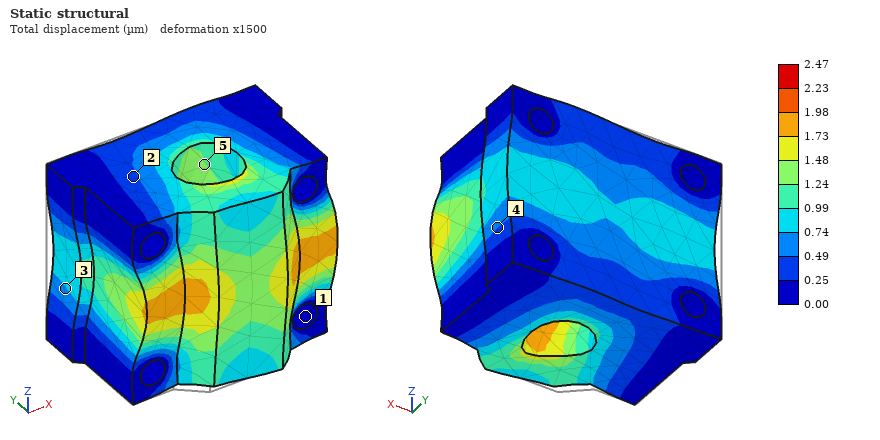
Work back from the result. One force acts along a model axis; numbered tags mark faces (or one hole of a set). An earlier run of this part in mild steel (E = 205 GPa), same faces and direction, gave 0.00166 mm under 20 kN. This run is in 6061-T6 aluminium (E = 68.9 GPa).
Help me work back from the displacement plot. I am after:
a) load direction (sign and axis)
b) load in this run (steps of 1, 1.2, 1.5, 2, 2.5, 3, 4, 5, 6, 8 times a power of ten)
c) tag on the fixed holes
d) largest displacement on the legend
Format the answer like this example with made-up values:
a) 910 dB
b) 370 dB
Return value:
a) +X
b) 10 kN
c) 1
d) 2.47 µm
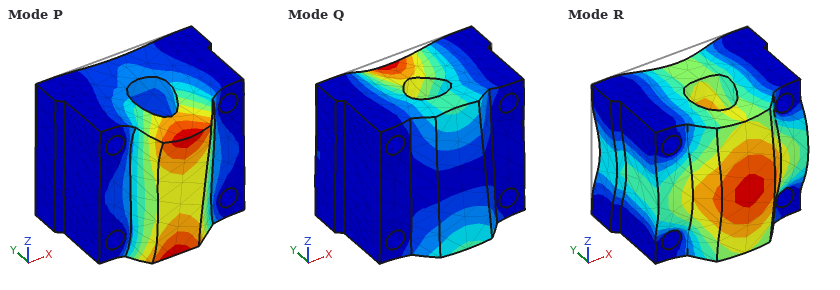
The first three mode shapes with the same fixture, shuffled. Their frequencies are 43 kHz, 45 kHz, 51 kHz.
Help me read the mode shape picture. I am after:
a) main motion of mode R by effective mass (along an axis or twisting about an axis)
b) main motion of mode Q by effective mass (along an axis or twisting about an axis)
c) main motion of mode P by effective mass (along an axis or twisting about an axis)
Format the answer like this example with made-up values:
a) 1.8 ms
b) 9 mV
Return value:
a) along Y
b) along Z
c) along Z
